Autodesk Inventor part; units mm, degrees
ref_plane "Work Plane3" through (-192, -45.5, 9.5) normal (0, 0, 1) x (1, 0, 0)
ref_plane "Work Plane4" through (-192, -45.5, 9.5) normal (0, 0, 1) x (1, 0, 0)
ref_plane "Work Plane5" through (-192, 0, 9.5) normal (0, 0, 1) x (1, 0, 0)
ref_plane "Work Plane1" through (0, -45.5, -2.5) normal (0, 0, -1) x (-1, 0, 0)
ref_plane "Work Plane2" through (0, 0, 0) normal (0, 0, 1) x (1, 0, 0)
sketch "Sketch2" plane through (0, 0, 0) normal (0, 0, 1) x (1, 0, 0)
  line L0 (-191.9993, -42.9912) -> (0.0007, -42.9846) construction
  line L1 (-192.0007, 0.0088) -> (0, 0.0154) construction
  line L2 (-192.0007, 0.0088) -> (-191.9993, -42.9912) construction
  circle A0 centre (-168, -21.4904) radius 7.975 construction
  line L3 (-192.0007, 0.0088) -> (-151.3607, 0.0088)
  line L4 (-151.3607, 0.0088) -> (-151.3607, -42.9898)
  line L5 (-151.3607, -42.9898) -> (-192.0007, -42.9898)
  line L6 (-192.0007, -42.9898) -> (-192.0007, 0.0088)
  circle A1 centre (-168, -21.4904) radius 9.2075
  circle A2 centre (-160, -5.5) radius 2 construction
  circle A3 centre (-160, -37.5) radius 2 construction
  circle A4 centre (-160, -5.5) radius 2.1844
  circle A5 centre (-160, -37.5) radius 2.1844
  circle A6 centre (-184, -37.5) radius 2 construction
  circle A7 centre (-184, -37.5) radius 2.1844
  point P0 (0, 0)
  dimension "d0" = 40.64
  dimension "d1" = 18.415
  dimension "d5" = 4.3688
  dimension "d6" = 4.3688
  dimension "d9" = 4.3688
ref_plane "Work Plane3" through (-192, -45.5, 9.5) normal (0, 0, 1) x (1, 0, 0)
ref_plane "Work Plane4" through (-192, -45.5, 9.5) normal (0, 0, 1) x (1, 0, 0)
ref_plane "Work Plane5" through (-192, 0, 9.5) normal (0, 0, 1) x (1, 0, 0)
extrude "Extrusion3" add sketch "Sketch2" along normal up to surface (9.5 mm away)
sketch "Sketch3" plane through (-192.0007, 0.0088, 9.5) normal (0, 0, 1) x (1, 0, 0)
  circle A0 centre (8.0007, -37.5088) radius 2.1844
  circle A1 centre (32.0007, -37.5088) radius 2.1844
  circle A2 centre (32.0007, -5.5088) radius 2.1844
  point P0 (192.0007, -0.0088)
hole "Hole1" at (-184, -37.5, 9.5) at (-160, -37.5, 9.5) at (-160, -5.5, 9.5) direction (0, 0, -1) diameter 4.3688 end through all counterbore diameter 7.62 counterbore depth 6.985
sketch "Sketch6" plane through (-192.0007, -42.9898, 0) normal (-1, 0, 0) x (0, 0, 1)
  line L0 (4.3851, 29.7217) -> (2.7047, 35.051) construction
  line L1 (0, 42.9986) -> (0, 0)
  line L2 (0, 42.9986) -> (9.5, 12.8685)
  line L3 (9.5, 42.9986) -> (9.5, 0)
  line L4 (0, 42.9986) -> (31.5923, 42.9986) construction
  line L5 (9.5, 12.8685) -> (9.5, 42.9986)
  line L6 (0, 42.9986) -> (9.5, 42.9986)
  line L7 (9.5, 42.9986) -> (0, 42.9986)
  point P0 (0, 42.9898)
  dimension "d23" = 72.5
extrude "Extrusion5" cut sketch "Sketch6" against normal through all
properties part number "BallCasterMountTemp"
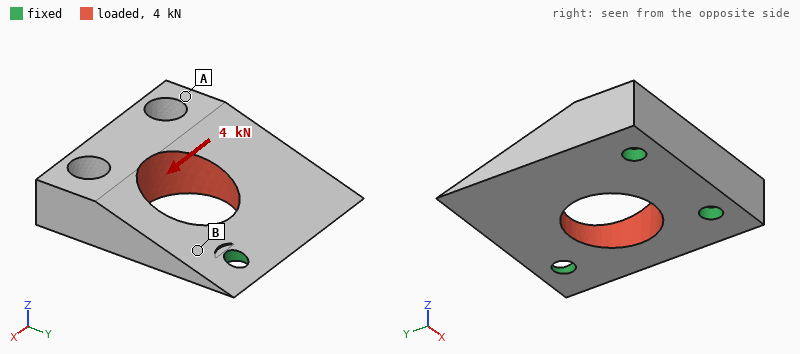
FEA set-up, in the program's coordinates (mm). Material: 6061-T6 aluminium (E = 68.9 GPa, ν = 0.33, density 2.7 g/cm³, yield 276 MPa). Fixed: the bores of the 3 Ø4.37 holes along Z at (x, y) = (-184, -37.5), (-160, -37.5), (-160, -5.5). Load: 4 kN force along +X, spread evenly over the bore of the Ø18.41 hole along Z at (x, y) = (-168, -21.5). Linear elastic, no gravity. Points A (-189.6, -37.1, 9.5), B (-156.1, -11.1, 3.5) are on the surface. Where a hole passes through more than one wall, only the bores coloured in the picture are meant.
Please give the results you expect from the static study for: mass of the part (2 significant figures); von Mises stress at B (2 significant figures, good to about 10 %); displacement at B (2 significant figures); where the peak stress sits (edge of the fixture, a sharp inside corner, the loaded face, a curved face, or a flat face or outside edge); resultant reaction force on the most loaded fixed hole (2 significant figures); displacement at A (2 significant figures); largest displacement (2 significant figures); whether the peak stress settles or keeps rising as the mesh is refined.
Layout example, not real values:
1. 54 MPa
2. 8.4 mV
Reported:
1. 22 g
2. 30 MPa
3. 6.7 µm
4. edge of the fixture
5. 1.5 kN
6. 6.1 µm
7. 14 µm
8. keeps rising
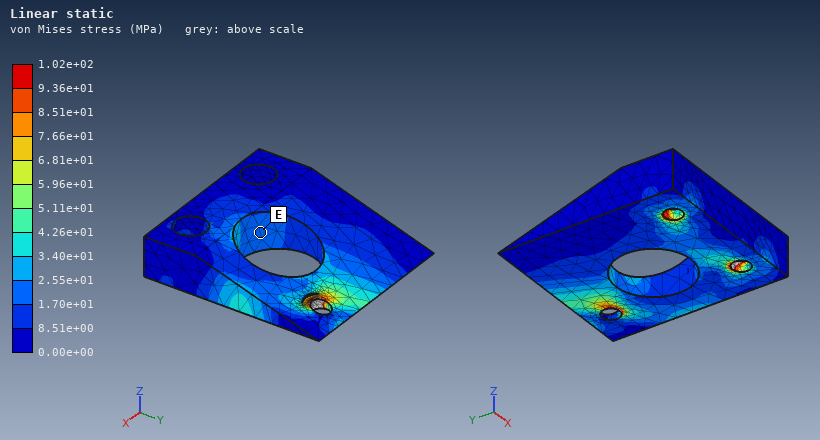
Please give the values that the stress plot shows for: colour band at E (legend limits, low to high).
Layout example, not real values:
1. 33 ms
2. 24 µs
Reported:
1. 1.70e+01 to 2.55e+01 MPa
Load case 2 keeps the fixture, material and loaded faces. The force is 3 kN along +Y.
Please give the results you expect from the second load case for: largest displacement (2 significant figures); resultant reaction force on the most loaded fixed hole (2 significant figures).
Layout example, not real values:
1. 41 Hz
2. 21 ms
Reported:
1. 27 µm
2. 1.2 kN
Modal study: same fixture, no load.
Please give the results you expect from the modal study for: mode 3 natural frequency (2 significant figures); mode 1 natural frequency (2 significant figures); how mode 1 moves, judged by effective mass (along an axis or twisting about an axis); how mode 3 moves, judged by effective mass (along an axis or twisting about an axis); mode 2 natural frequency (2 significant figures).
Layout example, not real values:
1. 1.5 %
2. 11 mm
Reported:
1. 19 kHz
2. 6700 Hz
3. along Z
4. twisting about Y
5. 17 kHz
